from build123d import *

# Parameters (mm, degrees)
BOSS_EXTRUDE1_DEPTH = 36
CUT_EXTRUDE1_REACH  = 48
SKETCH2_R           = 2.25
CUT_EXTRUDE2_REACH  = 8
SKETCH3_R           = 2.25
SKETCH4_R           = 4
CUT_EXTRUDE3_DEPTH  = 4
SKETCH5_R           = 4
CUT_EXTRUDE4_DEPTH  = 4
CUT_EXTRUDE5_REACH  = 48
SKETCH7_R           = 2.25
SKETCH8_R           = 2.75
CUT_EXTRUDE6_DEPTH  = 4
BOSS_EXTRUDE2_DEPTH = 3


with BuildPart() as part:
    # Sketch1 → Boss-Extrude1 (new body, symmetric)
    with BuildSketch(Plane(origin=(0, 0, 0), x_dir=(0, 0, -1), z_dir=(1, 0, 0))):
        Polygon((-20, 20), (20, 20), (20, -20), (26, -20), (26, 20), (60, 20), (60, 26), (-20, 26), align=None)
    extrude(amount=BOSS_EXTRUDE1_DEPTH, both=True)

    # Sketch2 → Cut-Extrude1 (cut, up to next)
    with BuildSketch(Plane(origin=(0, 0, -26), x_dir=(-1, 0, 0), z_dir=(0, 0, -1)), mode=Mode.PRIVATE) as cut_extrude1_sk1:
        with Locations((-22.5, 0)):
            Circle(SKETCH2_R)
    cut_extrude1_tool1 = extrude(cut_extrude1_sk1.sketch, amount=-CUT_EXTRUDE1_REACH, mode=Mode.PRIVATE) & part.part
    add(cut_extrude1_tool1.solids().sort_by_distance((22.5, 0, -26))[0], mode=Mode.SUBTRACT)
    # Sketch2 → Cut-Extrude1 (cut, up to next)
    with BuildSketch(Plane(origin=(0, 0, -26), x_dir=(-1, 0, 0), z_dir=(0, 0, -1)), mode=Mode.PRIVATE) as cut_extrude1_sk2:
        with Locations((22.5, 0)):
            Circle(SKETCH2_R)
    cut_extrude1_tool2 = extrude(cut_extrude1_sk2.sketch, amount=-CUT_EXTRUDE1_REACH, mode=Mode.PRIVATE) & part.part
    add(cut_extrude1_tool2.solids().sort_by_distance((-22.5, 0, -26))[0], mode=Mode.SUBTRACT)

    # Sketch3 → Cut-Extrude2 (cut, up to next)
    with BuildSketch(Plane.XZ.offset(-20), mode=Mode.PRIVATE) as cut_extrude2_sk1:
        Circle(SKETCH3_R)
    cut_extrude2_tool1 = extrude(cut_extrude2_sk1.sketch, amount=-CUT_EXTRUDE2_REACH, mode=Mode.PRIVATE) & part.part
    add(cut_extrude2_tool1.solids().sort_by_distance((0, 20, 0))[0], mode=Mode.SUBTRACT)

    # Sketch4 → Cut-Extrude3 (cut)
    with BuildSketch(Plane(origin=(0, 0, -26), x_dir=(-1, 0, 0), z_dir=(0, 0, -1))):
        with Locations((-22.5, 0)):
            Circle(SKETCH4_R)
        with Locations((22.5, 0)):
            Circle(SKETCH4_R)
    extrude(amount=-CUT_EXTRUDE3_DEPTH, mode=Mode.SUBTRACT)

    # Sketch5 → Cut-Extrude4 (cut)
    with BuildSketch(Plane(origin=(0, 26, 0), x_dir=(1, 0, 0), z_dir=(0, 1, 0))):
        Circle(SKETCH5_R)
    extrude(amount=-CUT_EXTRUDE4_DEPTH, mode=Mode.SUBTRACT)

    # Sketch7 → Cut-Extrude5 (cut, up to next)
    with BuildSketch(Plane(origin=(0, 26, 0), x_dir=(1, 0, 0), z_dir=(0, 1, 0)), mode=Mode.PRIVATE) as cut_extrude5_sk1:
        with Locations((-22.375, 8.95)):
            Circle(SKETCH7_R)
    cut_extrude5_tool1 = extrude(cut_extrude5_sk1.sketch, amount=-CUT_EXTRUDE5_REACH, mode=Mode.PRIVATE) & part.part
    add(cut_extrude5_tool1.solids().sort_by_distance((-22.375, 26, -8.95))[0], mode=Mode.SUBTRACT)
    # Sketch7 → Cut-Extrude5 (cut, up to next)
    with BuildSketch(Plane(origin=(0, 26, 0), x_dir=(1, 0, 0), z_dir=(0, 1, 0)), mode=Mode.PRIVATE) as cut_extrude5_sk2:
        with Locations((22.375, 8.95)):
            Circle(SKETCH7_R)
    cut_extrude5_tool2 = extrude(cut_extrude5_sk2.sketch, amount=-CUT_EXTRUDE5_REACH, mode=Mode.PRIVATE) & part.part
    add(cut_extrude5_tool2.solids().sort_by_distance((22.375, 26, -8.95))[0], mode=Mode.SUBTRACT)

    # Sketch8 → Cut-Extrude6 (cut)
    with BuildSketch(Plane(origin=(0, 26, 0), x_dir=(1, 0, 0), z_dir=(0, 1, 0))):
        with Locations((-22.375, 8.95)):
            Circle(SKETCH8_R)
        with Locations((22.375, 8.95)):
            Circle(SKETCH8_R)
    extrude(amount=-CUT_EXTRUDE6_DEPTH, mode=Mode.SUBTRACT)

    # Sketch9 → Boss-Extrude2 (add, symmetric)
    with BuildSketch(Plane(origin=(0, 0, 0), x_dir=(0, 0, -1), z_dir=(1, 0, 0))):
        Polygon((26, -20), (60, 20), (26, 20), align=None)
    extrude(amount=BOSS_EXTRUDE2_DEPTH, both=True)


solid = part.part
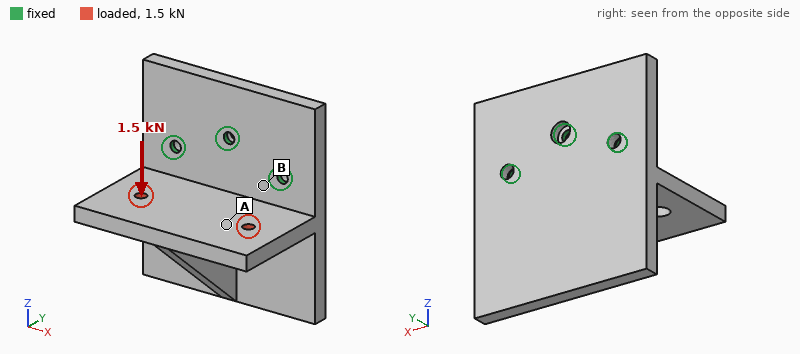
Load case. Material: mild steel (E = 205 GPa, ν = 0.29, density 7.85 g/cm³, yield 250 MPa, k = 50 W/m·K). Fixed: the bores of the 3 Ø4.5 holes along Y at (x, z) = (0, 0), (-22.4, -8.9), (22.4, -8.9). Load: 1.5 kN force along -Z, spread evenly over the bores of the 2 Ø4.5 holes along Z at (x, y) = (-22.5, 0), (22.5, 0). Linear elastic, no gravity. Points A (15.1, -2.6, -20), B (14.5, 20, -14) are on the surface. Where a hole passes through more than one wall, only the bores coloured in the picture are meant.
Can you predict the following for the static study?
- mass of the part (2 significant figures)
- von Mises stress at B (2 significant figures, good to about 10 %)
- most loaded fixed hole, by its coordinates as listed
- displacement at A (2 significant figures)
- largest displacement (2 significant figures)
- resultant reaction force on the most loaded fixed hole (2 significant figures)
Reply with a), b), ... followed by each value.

a) 430 g
b) 77 MPa
c) (0, 0)
d) 0.084 mm
e) 0.15 mm
f) 1.5 kN
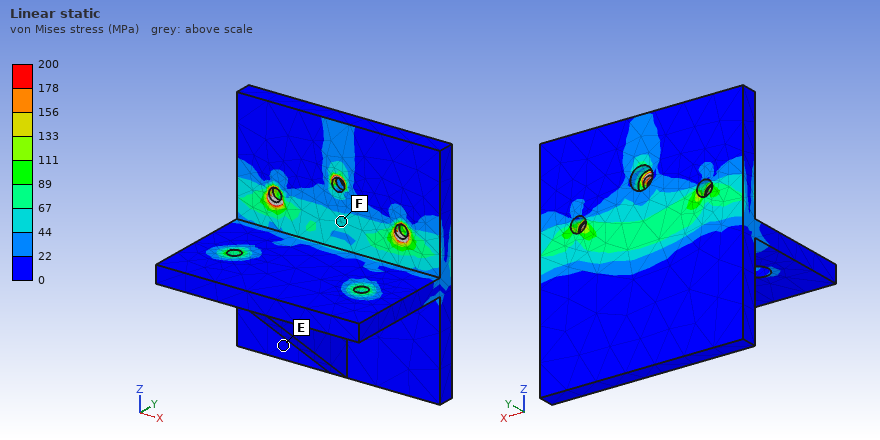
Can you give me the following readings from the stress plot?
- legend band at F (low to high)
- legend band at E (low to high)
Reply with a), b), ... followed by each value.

a) 44 to 67 MPa
b) 0 to 22 MPa
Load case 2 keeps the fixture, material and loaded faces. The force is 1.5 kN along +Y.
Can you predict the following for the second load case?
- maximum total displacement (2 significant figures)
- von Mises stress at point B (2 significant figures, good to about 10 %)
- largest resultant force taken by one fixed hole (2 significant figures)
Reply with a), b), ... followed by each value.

a) 62 µm
b) 27 MPa
c) 1.1 kN
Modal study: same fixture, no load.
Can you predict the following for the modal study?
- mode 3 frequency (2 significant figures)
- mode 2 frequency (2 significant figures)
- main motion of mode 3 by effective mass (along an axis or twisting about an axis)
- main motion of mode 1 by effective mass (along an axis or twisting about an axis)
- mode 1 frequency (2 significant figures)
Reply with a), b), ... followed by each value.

a) 4400 Hz
b) 3000 Hz
c) along Z
d) along Y
e) 1000 Hz
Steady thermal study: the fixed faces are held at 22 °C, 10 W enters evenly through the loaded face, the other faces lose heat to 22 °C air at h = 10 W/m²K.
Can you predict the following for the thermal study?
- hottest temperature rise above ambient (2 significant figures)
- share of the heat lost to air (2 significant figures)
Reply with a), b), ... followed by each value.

a) 25 K
b) 19 %
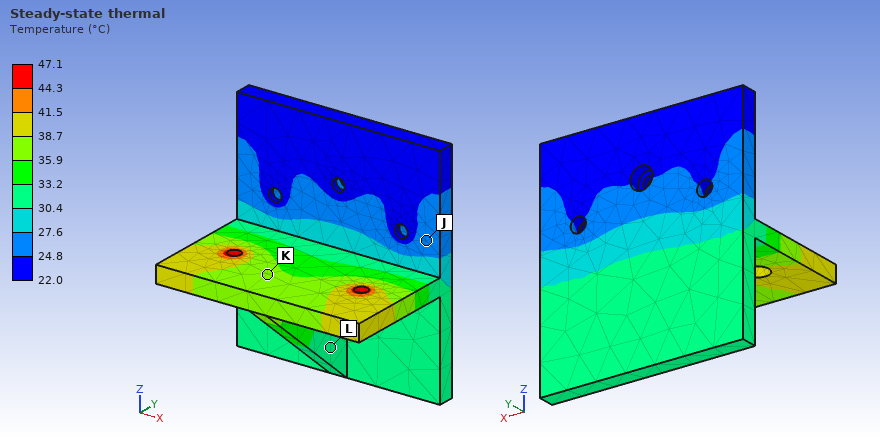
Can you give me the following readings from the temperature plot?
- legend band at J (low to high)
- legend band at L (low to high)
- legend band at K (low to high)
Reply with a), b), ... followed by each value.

a) 24.8 to 27.6 °C
b) 30.4 to 33.2 °C
c) 35.9 to 38.7 °C
